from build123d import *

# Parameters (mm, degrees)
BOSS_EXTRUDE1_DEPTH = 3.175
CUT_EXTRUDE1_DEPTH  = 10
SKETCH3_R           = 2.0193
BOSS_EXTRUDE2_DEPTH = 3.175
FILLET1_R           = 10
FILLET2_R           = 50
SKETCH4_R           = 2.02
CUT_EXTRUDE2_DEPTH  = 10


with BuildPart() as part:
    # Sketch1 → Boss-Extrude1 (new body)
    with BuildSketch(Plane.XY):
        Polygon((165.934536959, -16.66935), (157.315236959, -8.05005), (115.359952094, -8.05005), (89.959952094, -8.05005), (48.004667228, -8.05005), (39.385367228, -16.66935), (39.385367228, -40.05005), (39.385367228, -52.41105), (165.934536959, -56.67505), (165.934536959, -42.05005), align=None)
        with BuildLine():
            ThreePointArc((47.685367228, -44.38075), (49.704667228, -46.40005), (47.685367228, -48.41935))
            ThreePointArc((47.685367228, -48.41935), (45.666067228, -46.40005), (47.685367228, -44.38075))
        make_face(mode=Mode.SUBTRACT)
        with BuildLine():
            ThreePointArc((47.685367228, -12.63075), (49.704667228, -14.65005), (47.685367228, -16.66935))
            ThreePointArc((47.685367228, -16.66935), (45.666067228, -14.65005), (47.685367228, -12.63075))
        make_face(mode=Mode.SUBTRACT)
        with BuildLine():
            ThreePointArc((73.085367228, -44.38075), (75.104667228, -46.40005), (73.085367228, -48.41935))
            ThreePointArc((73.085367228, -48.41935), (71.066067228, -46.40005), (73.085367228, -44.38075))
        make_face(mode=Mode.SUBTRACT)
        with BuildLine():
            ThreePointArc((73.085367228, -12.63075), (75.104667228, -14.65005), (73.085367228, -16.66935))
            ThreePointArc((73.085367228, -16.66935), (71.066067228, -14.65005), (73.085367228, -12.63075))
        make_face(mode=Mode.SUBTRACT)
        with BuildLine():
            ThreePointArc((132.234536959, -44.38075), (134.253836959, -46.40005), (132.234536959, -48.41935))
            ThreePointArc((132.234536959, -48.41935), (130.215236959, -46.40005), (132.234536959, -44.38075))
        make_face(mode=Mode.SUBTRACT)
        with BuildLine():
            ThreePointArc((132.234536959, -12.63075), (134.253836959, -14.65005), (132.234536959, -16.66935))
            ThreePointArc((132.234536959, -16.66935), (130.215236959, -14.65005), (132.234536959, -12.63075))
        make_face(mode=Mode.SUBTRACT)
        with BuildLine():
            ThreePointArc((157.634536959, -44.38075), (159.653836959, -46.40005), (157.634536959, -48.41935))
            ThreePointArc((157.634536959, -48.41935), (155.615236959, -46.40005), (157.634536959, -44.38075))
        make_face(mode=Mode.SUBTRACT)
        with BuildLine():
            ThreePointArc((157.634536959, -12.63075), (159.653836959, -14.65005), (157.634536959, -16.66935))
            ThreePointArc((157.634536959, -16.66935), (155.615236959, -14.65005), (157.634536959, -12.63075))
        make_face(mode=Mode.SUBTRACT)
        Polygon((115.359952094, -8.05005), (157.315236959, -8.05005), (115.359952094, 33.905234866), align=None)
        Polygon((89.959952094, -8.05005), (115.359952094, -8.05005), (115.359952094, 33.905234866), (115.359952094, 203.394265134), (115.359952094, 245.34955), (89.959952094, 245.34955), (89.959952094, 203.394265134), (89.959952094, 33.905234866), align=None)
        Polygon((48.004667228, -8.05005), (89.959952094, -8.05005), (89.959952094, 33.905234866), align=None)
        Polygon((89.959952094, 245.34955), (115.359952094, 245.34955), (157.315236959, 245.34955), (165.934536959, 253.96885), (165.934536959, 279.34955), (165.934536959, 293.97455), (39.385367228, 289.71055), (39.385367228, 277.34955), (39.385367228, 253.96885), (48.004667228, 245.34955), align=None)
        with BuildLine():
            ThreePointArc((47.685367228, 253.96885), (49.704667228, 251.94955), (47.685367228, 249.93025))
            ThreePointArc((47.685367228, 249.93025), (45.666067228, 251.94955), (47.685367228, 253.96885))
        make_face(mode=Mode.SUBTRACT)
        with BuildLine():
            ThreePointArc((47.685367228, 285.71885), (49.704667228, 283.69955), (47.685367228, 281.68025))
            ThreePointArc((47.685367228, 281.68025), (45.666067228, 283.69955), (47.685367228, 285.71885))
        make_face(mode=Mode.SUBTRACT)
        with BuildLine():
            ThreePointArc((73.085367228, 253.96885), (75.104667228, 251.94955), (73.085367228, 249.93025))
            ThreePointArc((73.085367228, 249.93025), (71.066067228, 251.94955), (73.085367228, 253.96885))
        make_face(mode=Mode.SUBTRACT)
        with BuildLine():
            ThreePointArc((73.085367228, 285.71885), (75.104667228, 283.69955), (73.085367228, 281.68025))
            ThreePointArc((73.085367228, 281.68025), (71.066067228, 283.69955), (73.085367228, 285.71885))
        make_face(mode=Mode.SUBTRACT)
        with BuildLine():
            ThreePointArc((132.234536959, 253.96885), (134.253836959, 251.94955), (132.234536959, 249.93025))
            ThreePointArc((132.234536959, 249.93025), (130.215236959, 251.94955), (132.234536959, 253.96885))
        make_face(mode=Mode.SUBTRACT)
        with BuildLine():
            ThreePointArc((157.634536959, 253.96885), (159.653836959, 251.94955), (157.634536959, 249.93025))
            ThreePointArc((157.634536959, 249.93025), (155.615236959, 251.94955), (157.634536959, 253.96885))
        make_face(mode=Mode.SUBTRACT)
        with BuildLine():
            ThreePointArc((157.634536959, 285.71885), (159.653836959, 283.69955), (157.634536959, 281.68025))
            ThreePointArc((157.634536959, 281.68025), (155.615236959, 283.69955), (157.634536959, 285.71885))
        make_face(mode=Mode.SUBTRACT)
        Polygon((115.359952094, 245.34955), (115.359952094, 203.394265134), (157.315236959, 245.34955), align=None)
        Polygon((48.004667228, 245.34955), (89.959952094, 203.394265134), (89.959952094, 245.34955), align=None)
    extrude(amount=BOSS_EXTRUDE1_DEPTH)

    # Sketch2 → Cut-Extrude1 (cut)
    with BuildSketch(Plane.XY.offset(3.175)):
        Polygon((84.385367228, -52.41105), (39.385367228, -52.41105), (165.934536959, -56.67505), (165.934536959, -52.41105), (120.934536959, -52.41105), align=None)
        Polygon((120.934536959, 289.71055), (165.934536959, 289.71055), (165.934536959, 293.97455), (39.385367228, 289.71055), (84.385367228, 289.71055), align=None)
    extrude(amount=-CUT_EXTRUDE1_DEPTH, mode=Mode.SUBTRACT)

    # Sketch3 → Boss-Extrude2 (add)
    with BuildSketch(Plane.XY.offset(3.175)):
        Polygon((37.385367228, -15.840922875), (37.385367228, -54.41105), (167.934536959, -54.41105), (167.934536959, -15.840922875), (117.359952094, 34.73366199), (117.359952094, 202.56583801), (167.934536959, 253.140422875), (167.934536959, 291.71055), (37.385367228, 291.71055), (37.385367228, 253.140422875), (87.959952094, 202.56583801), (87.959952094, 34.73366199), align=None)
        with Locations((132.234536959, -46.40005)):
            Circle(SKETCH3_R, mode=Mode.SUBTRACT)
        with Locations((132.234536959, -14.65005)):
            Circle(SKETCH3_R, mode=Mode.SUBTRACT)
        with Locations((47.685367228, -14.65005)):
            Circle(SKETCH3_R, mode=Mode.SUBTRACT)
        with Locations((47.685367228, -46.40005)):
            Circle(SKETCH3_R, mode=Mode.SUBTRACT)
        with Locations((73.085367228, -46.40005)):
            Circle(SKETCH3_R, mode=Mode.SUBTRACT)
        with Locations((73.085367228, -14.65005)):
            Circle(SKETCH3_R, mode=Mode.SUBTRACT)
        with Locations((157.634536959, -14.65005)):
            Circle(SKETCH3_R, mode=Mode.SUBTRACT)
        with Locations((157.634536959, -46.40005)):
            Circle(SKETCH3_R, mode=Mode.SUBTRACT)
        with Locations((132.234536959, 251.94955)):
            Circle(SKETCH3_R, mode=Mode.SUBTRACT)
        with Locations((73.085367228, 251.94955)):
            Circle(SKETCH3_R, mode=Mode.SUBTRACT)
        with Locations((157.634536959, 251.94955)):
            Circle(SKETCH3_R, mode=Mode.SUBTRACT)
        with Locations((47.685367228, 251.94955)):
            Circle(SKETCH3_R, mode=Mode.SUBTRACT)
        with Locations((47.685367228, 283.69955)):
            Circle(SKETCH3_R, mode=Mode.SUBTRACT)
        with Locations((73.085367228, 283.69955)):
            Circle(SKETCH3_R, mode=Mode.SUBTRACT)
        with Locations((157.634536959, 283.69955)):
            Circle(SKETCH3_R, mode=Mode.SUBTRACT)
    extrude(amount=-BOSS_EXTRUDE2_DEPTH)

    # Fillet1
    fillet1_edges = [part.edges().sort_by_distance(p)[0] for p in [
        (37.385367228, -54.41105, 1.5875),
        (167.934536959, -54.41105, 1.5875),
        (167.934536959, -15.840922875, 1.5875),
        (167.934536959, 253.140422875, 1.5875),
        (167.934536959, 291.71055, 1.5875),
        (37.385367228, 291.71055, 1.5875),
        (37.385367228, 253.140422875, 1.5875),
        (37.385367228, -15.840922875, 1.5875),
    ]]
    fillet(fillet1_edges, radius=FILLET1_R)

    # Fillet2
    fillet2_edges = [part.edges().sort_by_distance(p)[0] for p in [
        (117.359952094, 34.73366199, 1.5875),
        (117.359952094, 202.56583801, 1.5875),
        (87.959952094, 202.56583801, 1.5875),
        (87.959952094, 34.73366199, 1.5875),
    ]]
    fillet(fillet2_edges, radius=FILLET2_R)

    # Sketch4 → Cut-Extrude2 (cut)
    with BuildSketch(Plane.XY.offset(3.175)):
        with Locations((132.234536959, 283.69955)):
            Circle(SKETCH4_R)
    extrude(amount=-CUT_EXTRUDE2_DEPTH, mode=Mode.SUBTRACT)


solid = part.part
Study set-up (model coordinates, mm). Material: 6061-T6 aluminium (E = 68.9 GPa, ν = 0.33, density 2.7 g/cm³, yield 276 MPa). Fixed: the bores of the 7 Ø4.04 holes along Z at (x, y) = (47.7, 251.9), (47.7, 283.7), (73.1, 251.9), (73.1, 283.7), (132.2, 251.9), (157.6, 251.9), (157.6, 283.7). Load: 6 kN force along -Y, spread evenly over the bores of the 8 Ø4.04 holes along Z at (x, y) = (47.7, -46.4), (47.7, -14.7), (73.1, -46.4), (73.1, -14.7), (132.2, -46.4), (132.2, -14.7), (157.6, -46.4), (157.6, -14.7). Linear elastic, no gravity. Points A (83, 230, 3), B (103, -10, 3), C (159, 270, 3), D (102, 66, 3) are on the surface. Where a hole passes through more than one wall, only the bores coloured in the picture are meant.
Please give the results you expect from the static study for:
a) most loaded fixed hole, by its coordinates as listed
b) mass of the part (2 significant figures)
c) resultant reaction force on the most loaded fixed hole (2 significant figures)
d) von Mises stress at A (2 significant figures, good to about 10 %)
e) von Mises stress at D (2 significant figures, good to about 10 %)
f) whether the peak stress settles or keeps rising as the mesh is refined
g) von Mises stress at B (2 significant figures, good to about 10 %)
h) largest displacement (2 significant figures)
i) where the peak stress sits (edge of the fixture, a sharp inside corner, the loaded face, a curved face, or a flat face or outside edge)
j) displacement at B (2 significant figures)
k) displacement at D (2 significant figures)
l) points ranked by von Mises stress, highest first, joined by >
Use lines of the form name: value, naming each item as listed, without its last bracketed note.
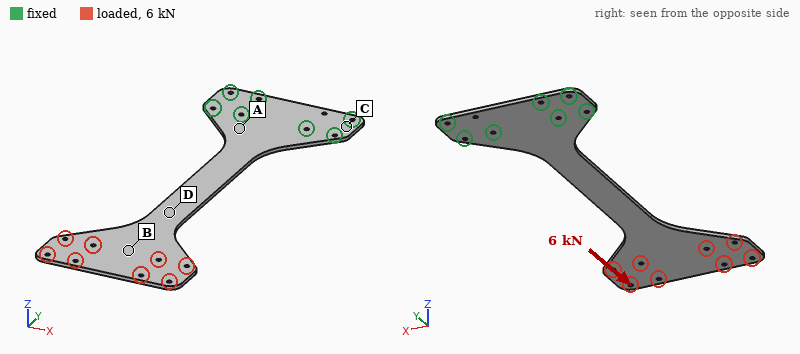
most loaded fixed hole, by its coordinates as listed: (132.2, 251.9)
mass of the part: 200 g
resultant reaction force on the most loaded fixed hole: 2.2 kN
von Mises stress at A: 32 MPa
von Mises stress at D: 64 MPa
whether the peak stress settles or keeps rising as the mesh is refined: keeps rising
von Mises stress at B: 18 MPa
largest displacement: 0.23 mm
where the peak stress sits: edge of the fixture
displacement at B: 0.20 mm
displacement at D: 0.16 mm
points ranked by von Mises stress, highest first, joined by >: D > A > B > C
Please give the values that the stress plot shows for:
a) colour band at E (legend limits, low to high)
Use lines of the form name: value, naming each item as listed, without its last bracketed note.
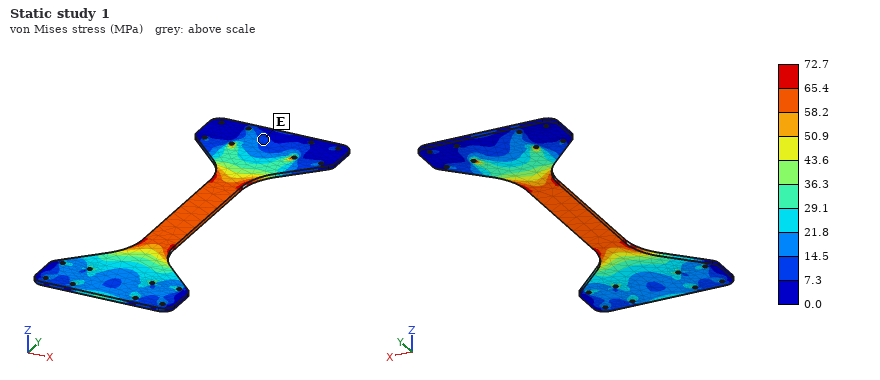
colour band at E: 7.3 to 14.5 MPa
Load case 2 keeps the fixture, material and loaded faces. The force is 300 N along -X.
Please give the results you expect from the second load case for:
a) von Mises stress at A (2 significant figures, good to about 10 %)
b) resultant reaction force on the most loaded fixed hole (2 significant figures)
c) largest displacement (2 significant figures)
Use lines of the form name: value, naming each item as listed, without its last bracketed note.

von Mises stress at A: 21 MPa
resultant reaction force on the most loaded fixed hole: 760 N
largest displacement: 3.4 mm
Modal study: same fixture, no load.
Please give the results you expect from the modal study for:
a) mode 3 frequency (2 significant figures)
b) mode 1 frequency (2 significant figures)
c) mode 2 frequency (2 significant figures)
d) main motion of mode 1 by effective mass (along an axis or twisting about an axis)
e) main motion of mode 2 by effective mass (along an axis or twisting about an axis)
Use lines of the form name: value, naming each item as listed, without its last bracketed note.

mode 3 frequency: 170 Hz
mode 1 frequency: 18 Hz
mode 2 frequency: 110 Hz
main motion of mode 1 by effective mass: along Z
main motion of mode 2 by effective mass: twisting about Y
